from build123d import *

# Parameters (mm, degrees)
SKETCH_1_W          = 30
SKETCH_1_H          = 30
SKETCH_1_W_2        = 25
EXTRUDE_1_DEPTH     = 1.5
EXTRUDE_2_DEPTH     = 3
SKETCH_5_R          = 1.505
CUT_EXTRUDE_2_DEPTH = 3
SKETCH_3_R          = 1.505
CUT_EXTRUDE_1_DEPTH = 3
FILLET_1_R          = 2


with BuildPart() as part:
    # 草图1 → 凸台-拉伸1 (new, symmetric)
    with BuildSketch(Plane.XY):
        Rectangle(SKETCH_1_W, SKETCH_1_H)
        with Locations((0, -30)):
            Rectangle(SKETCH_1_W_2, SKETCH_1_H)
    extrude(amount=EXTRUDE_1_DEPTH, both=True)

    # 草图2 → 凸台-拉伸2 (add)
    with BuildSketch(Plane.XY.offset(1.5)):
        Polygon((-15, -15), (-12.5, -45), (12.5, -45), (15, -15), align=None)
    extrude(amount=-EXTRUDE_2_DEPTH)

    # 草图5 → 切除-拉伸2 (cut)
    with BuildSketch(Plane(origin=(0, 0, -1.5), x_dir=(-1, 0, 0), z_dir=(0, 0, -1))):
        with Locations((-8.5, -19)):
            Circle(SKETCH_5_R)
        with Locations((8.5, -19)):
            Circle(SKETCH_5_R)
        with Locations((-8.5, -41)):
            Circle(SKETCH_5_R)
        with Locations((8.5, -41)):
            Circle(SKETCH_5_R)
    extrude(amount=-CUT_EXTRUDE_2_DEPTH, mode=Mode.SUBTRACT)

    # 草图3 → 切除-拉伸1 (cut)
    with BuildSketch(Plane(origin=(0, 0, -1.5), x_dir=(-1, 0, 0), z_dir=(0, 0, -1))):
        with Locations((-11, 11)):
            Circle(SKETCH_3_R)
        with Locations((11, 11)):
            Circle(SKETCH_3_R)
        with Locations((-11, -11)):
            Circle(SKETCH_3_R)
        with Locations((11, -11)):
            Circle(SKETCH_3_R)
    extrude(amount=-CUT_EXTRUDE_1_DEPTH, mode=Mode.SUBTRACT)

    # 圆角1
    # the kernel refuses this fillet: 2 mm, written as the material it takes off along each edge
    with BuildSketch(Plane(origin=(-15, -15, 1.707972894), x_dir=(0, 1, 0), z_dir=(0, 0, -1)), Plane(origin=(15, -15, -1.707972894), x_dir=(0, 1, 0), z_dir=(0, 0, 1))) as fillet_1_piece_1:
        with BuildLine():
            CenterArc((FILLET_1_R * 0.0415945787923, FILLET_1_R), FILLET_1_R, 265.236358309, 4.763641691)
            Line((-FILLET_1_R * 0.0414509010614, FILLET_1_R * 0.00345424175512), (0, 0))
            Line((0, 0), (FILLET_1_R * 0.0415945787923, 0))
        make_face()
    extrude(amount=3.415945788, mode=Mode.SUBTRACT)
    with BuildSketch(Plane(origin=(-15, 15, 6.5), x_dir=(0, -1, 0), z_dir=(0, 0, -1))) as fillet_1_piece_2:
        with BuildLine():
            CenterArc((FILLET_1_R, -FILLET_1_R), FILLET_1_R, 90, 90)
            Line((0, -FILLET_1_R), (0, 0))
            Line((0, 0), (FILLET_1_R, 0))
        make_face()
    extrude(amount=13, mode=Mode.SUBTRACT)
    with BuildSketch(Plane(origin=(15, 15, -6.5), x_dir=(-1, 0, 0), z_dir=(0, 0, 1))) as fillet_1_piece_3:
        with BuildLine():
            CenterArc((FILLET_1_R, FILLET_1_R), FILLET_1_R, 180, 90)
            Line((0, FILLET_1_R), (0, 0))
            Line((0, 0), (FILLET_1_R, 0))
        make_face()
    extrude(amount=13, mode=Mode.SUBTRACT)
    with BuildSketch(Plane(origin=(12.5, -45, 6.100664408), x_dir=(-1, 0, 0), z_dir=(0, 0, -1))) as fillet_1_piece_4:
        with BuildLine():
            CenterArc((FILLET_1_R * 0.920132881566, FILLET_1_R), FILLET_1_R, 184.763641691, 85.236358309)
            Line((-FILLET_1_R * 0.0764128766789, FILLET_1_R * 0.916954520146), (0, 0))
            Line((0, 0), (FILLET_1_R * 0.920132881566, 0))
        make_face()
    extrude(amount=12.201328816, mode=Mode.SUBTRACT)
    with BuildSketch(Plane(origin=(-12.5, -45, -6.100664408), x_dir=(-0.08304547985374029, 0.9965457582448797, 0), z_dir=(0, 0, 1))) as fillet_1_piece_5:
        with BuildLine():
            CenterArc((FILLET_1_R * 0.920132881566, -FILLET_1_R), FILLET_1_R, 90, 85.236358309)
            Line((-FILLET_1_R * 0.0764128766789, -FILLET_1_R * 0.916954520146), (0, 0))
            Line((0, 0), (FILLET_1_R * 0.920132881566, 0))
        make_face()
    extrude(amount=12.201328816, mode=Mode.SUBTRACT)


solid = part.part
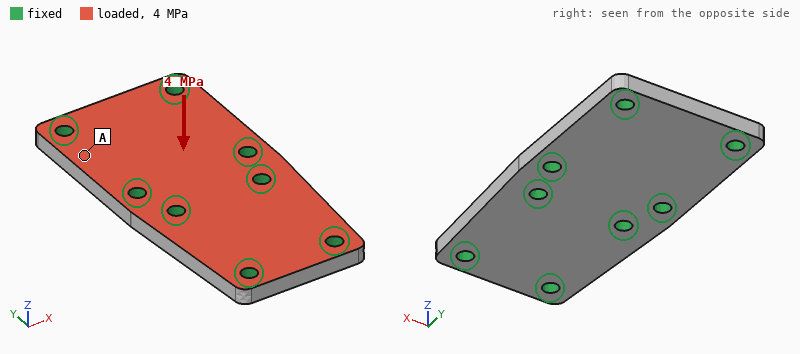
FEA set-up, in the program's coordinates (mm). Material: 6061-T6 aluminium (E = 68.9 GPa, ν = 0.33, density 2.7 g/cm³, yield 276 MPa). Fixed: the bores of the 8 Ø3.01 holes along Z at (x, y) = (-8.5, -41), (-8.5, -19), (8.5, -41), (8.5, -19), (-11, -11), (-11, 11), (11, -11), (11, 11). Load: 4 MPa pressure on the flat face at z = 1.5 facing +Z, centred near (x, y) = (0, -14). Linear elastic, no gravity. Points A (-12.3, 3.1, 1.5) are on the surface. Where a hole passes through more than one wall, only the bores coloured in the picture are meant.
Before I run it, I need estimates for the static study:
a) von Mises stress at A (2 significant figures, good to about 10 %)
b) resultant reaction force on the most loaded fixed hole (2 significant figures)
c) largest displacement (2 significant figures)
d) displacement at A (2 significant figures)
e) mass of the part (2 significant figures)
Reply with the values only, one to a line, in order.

41 MPa
900 N
34 µm
15 µm
13 g
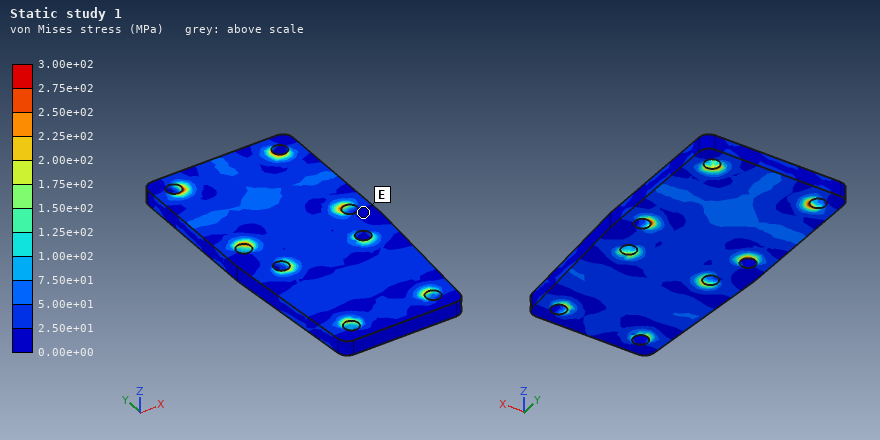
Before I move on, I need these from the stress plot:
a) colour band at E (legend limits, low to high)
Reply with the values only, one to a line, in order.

0.00e+00 to 2.50e+01 MPa
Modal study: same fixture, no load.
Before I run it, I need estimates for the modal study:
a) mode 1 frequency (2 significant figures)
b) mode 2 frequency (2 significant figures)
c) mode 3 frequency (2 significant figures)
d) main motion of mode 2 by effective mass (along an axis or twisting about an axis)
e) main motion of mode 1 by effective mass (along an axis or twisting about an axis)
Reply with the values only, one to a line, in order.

23 kHz
28 kHz
33 kHz
along Z
along Z
